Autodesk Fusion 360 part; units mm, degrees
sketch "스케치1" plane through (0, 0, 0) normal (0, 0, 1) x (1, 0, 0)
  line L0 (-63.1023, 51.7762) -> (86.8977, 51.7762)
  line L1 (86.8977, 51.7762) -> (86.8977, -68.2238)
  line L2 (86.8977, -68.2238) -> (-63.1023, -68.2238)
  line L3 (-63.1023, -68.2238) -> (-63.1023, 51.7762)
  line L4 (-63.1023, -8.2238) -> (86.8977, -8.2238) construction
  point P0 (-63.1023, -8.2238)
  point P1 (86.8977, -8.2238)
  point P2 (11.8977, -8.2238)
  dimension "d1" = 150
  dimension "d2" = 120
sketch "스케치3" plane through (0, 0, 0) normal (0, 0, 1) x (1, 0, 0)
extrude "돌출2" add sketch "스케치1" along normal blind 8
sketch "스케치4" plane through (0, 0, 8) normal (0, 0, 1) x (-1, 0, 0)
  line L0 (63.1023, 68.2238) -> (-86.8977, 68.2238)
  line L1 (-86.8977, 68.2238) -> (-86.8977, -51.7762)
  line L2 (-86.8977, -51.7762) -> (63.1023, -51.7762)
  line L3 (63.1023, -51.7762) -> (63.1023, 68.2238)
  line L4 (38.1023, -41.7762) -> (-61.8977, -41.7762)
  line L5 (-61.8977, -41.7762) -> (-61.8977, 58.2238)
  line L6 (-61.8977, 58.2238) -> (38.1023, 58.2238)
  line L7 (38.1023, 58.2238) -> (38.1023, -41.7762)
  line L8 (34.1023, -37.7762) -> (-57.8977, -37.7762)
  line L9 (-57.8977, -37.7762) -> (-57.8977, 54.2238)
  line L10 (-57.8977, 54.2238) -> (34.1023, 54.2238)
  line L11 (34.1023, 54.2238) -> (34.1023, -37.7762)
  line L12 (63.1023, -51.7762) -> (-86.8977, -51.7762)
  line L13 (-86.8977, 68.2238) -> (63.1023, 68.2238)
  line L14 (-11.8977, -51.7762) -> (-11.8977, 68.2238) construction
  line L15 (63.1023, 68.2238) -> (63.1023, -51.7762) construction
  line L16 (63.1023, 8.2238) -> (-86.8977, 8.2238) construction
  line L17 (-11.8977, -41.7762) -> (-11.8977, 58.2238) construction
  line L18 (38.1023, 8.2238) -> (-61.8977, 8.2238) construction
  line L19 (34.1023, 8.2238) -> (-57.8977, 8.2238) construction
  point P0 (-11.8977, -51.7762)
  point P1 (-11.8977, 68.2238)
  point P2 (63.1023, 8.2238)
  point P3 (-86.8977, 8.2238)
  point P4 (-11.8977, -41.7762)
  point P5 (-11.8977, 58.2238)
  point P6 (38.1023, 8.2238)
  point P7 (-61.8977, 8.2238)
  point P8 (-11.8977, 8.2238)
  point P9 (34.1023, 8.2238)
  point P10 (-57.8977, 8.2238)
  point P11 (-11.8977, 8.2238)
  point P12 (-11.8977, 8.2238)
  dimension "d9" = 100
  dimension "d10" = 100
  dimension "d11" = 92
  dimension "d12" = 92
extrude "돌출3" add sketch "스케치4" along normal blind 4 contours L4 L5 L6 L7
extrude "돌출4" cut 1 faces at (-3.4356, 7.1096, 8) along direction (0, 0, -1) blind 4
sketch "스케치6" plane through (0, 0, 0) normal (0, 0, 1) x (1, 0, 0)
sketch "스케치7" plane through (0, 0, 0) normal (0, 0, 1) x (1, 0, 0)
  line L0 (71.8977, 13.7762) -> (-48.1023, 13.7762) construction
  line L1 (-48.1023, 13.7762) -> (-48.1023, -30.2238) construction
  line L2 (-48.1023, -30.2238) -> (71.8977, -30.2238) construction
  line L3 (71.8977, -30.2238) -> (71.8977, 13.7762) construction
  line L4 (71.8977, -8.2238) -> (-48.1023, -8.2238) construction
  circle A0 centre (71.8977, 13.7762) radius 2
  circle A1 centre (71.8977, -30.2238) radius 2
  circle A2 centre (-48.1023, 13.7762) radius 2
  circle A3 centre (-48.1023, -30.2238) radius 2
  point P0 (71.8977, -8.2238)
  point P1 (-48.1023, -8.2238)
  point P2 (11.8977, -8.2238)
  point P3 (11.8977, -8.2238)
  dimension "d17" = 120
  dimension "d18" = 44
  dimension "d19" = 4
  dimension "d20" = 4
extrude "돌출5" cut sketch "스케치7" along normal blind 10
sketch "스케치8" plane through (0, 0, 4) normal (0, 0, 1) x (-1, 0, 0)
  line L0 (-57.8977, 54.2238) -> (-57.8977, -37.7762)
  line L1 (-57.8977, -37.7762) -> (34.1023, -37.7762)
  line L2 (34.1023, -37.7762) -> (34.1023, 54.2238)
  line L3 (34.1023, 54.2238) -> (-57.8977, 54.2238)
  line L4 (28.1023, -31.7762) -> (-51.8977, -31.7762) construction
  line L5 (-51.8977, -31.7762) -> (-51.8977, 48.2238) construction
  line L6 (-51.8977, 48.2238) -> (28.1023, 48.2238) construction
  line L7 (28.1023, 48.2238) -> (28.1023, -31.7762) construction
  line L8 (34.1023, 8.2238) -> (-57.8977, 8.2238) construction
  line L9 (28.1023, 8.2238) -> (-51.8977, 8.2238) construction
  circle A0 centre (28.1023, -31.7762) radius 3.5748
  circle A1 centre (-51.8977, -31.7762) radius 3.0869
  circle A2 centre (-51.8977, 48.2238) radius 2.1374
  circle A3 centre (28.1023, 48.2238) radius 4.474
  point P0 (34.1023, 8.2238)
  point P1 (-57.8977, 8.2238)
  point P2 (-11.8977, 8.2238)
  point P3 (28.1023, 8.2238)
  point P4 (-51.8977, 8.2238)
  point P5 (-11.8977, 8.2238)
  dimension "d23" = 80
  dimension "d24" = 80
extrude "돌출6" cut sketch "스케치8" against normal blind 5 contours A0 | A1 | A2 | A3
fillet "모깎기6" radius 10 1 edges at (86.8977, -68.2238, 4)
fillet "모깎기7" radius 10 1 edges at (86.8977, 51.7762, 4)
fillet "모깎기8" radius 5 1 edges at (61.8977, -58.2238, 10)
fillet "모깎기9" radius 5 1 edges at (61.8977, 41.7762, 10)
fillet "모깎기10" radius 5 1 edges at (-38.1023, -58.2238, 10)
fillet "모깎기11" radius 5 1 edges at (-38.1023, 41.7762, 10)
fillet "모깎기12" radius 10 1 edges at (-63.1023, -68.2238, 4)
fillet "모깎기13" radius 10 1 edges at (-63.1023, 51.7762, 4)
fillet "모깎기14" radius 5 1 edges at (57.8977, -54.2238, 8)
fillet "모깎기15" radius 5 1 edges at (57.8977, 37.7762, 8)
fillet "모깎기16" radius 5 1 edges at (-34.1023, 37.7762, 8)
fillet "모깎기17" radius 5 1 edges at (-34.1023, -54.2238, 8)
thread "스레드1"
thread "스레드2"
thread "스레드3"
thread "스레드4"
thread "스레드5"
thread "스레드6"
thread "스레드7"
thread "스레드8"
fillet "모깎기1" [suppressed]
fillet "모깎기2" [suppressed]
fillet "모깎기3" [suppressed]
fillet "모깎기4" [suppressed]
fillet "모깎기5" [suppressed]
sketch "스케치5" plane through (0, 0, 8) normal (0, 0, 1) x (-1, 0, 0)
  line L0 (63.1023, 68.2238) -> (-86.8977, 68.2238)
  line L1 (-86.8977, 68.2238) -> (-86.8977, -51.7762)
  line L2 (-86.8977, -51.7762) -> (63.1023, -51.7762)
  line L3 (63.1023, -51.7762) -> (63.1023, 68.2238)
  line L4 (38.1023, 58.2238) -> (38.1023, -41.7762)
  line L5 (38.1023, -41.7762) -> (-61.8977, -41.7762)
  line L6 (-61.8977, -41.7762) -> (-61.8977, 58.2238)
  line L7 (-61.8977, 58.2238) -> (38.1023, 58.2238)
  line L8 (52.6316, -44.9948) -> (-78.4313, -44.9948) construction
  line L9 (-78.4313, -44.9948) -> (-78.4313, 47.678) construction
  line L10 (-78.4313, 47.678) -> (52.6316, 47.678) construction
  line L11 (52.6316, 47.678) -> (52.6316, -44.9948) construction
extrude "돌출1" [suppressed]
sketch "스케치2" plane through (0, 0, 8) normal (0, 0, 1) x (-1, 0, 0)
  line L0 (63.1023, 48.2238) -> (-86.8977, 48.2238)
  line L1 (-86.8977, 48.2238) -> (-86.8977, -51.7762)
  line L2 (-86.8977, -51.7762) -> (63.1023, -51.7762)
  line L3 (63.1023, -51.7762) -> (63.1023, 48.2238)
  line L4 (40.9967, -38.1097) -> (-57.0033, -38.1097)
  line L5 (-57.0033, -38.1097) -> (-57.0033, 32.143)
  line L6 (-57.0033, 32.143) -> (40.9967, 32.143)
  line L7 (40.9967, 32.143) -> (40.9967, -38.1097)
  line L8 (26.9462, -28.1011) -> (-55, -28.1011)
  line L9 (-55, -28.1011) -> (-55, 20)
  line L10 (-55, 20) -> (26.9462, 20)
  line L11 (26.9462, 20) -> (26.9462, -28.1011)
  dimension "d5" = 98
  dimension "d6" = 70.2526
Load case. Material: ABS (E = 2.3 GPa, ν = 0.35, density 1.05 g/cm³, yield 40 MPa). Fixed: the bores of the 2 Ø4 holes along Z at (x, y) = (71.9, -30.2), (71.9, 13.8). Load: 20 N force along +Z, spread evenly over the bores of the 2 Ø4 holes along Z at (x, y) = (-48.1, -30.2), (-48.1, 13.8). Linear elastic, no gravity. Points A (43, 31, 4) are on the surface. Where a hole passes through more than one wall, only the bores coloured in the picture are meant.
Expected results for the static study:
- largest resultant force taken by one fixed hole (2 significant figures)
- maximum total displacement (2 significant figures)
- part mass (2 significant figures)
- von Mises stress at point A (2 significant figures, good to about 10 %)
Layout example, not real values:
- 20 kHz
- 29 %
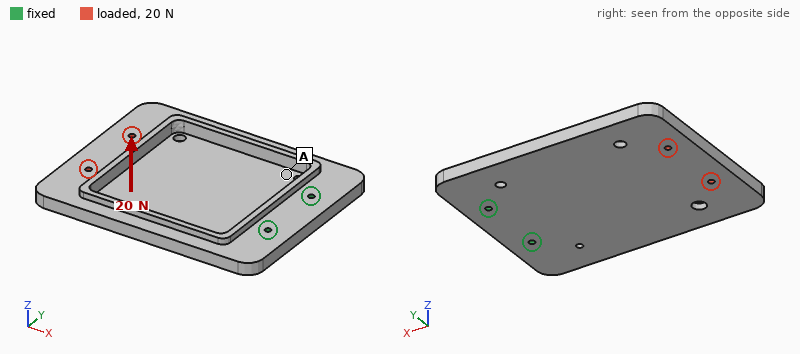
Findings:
- 25 N
- 2.3 mm
- 120 g
- 0.75 MPa
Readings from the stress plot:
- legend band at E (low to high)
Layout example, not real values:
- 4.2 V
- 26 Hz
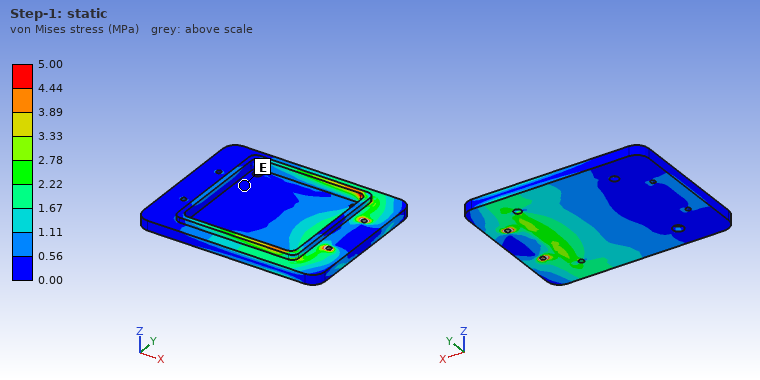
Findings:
- 0.00 to 0.56 MPa
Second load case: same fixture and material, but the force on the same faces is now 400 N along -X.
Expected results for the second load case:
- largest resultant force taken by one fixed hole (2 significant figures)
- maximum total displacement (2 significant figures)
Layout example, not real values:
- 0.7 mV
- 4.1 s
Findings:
- 200 N
- 0.66 mm
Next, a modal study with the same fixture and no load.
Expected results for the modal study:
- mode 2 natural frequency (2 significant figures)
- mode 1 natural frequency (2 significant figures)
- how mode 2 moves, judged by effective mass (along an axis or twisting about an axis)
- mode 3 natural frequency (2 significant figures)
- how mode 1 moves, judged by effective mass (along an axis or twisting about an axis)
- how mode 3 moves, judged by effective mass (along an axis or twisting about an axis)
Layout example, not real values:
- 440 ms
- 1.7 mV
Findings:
- 180 Hz
- 79 Hz
- twisting about X
- 520 Hz
- along Z
- along Z
